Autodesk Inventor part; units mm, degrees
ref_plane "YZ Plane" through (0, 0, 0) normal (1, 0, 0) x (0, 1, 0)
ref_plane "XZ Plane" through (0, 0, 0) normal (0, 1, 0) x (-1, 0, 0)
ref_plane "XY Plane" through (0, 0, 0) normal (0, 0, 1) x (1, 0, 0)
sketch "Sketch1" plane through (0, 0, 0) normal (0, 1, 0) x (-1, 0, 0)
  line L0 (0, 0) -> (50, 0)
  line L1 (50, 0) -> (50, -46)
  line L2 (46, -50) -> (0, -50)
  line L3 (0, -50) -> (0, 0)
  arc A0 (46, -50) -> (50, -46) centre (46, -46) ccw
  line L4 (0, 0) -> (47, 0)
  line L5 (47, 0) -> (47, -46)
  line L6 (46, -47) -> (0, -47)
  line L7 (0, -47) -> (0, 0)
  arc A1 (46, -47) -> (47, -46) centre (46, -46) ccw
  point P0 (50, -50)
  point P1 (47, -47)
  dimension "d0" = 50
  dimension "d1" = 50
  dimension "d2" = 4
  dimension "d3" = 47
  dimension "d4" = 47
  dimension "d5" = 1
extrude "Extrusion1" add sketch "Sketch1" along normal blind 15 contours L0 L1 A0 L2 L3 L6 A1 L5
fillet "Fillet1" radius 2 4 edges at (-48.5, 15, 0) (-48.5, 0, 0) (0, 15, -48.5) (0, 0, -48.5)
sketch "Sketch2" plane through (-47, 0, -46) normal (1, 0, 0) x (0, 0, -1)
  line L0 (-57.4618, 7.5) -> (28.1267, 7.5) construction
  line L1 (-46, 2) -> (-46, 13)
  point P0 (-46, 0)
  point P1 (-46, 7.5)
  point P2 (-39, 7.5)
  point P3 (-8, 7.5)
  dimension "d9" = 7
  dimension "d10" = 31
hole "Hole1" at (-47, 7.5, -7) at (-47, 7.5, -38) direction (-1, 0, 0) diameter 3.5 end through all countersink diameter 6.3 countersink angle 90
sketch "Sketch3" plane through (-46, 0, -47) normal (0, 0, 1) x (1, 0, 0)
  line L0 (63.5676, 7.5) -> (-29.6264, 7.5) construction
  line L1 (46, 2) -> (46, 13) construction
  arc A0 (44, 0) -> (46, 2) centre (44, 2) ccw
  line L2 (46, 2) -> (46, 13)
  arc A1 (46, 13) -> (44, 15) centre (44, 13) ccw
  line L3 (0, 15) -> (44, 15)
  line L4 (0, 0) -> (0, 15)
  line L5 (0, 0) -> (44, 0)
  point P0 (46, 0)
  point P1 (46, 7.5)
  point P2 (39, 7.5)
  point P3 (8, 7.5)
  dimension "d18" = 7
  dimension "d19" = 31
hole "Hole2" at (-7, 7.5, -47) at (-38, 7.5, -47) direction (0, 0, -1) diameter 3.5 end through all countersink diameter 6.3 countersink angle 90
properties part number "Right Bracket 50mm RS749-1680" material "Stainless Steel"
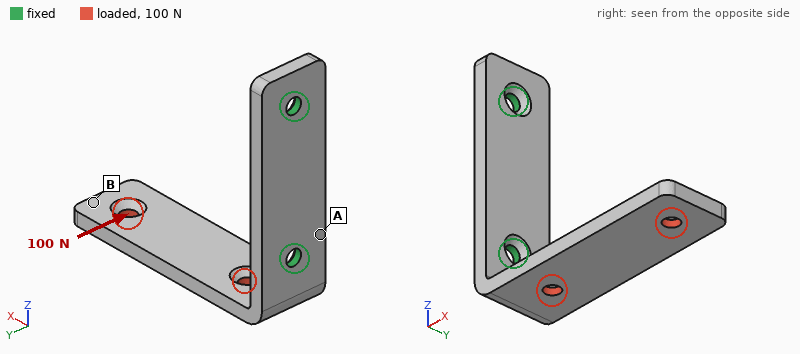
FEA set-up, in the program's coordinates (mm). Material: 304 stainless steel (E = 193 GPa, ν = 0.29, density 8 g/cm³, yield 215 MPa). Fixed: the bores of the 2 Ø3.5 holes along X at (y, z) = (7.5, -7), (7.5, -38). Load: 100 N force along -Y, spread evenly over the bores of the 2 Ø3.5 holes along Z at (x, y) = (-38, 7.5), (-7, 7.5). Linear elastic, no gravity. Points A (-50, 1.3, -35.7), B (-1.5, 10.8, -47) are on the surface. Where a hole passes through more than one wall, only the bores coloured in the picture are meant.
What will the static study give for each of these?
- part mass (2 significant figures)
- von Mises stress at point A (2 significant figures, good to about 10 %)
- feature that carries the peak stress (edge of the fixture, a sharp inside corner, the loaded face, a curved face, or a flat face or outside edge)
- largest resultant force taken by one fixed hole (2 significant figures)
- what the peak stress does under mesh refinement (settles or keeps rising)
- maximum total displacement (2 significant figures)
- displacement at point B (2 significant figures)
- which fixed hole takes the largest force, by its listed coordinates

33 g
57 MPa
edge of the fixture
120 N
keeps rising
0.17 mm
0.16 mm
(7.5, -38)
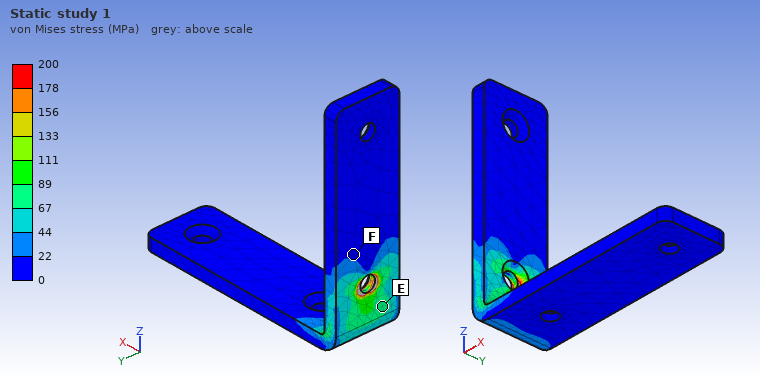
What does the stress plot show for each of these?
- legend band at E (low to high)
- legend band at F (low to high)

67 to 89 MPa
0 to 22 MPa
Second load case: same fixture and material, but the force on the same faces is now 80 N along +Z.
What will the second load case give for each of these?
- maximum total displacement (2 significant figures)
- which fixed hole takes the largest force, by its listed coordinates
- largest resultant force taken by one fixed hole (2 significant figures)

0.39 mm
(7.5, -7)
110 N
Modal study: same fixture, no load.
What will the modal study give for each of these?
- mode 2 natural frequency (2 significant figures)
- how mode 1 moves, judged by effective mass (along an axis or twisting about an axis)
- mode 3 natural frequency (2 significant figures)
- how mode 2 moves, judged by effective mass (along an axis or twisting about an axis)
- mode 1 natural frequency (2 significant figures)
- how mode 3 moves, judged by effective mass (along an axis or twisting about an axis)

1200 Hz
along Z
4200 Hz
along Y
730 Hz
along X
